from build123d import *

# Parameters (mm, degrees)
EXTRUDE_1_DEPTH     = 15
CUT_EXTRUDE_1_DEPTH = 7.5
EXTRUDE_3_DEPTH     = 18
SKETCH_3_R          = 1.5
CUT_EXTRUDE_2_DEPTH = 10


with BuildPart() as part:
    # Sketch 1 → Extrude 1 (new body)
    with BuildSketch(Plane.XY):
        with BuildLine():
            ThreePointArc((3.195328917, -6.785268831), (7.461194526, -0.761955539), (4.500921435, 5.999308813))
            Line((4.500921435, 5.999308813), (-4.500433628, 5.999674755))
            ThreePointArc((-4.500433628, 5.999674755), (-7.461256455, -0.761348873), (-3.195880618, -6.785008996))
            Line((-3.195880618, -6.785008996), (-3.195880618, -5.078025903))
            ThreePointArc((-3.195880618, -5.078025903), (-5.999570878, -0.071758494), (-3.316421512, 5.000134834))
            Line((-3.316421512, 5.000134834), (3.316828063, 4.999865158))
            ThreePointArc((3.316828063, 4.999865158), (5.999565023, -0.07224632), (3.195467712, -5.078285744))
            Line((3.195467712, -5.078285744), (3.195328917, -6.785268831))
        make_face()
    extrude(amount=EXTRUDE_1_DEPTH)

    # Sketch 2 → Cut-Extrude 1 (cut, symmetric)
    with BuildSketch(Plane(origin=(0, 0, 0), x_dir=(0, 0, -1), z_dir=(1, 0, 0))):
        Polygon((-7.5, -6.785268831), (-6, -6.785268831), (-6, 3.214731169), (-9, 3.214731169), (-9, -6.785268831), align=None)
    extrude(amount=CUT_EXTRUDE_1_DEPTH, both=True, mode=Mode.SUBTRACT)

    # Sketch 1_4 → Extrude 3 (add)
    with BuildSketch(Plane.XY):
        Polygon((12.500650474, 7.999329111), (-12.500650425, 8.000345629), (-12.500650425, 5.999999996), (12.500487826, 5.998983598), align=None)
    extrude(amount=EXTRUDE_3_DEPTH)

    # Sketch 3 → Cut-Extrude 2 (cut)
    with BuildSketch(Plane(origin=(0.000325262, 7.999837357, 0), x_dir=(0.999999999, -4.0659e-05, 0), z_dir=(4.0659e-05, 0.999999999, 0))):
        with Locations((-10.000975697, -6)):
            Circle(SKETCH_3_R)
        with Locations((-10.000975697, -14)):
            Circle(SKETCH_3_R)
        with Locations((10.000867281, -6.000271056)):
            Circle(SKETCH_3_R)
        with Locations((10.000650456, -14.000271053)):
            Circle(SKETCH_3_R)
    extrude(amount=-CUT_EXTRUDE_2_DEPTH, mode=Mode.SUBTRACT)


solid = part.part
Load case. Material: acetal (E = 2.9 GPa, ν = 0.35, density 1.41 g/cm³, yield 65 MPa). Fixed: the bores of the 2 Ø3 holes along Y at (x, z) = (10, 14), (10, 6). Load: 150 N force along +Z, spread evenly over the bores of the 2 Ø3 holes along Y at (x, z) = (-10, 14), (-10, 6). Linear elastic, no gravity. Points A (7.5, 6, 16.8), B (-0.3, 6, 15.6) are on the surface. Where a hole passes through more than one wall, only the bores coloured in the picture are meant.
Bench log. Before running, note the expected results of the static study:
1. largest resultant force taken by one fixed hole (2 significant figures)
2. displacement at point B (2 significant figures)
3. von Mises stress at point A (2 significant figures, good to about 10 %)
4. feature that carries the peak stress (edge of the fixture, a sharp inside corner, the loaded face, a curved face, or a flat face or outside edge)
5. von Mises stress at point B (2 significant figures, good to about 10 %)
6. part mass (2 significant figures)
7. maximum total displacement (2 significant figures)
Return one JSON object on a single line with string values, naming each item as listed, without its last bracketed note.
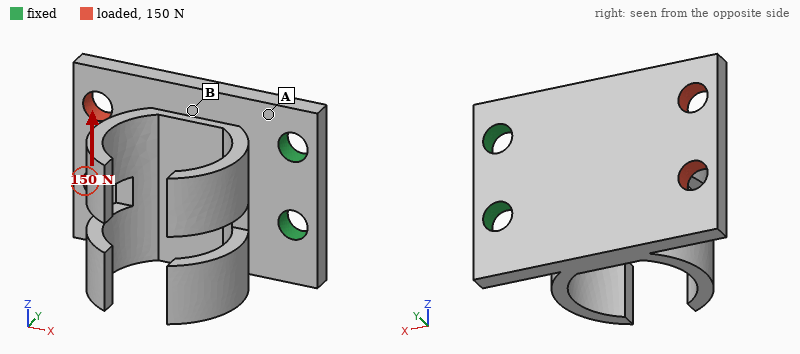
{"largest resultant force taken by one fixed hole": "290 N", "displacement at point B": "0.14 mm", "von Mises stress at point A": "21 MPa", "feature that carries the peak stress": "edge of the fixture", "von Mises stress at point B": "8.6 MPa", "part mass": "2.1 g", "maximum total displacement": "0.38 mm"}
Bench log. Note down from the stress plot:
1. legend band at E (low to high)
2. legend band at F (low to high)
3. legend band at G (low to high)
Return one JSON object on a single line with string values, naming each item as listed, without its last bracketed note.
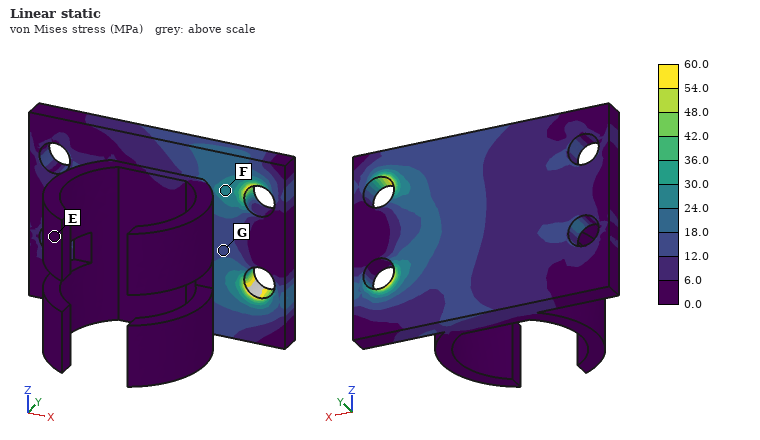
{"legend band at E": "0.0 to 6.0 MPa", "legend band at F": "24.0 to 30.0 MPa", "legend band at G": "12.0 to 18.0 MPa"}
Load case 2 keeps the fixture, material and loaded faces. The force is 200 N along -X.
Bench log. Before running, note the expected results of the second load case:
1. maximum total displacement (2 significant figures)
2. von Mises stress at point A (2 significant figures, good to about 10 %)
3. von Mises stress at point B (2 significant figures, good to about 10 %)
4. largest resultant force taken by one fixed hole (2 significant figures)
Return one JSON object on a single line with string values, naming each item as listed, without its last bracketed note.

{"maximum total displacement": "0.11 mm", "von Mises stress at point A": "4.9 MPa", "von Mises stress at point B": "3.9 MPa", "largest resultant force taken by one fixed hole": "100 N"}
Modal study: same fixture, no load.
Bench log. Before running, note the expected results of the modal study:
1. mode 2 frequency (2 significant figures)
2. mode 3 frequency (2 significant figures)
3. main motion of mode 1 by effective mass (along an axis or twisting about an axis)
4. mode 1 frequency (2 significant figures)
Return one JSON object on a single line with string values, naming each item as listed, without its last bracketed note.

{"mode 2 frequency": "1800 Hz", "mode 3 frequency": "2000 Hz", "main motion of mode 1 by effective mass": "along Y", "mode 1 frequency": "810 Hz"}
